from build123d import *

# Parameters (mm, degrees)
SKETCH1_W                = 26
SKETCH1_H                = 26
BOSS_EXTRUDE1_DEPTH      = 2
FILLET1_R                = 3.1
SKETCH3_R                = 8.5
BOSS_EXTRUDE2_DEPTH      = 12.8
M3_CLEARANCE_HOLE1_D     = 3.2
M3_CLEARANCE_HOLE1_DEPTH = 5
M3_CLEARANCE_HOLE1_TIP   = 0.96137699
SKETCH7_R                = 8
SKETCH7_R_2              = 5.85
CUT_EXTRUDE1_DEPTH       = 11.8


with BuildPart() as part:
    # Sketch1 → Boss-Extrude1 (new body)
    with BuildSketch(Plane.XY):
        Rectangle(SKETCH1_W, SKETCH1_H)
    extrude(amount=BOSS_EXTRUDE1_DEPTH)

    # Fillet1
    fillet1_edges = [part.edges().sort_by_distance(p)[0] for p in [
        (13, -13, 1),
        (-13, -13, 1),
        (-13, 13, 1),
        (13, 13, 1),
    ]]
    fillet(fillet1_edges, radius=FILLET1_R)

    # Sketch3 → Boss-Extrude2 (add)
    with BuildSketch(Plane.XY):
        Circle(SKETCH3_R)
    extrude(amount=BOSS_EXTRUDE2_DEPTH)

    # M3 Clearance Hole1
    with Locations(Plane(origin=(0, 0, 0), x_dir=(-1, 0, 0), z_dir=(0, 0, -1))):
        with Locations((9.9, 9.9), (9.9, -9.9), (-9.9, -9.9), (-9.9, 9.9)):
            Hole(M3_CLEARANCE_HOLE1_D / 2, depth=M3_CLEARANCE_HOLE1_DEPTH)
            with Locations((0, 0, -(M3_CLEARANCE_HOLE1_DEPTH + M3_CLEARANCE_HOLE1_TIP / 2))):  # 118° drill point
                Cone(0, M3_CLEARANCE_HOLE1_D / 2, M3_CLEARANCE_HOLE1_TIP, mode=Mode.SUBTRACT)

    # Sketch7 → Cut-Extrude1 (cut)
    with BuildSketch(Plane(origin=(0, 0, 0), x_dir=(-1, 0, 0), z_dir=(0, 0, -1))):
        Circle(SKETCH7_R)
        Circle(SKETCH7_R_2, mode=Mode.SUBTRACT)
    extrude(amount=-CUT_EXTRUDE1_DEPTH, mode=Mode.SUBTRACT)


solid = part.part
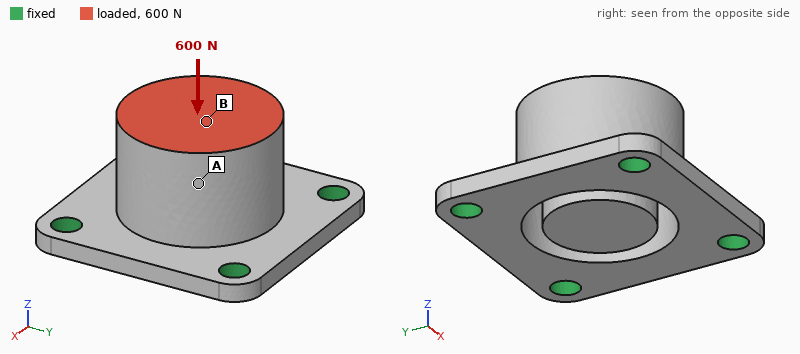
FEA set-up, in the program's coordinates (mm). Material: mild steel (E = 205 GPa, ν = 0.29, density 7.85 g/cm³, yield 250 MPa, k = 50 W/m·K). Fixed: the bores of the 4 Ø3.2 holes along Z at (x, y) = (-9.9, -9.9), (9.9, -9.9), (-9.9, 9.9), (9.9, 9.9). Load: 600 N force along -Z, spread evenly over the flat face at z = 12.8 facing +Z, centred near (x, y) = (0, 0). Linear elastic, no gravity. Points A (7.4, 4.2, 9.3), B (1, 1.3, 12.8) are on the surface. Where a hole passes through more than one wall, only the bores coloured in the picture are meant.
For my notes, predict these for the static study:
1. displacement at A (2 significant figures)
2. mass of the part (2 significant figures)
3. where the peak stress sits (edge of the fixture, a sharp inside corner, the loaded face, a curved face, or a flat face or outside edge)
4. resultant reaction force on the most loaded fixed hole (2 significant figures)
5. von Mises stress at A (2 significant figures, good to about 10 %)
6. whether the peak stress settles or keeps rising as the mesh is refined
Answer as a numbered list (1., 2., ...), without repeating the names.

1. 5.3 µm
2. 21 g
3. edge of the fixture
4. 150 N
5. 31 MPa
6. keeps rising
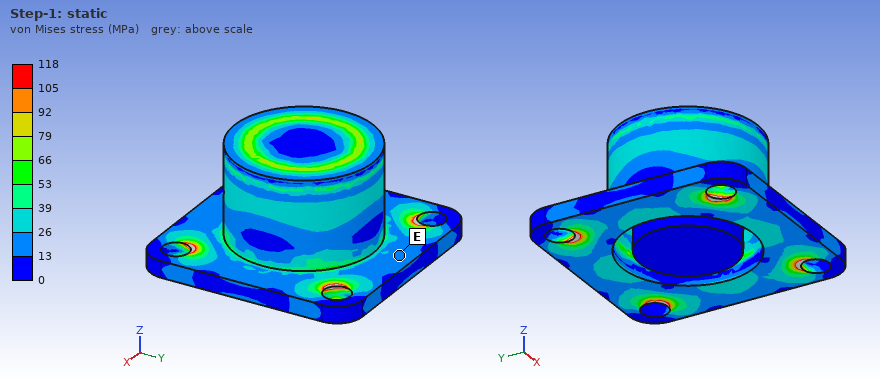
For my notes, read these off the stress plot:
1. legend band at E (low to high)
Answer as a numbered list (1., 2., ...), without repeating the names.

1. 13 to 26 MPa
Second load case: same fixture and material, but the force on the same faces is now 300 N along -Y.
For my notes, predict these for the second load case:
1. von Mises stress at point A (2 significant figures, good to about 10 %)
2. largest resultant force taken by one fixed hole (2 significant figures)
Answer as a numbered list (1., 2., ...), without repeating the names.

1. 35 MPa
2. 140 N
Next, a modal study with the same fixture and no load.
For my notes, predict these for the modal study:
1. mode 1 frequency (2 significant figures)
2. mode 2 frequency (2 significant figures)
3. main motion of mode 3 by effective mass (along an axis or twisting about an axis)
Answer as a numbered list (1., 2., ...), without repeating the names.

1. 8600 Hz
2. 8600 Hz
3. along Z
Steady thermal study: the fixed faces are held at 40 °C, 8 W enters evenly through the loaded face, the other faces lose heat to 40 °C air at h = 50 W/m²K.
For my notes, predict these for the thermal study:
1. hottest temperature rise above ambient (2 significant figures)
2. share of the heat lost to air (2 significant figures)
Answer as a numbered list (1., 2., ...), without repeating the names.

1. 55 K
2. 42 %
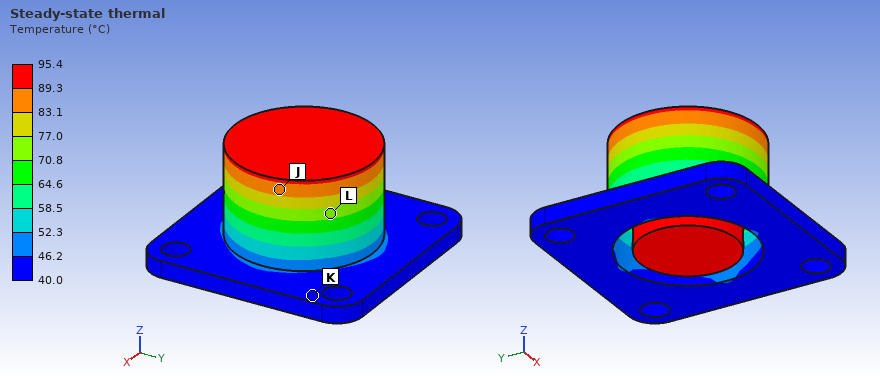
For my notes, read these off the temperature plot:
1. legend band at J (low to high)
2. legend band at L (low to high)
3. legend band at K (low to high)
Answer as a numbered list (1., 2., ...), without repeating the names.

1. 83.1 to 89.3 °C
2. 70.8 to 77.0 °C
3. 40.0 to 46.2 °C
